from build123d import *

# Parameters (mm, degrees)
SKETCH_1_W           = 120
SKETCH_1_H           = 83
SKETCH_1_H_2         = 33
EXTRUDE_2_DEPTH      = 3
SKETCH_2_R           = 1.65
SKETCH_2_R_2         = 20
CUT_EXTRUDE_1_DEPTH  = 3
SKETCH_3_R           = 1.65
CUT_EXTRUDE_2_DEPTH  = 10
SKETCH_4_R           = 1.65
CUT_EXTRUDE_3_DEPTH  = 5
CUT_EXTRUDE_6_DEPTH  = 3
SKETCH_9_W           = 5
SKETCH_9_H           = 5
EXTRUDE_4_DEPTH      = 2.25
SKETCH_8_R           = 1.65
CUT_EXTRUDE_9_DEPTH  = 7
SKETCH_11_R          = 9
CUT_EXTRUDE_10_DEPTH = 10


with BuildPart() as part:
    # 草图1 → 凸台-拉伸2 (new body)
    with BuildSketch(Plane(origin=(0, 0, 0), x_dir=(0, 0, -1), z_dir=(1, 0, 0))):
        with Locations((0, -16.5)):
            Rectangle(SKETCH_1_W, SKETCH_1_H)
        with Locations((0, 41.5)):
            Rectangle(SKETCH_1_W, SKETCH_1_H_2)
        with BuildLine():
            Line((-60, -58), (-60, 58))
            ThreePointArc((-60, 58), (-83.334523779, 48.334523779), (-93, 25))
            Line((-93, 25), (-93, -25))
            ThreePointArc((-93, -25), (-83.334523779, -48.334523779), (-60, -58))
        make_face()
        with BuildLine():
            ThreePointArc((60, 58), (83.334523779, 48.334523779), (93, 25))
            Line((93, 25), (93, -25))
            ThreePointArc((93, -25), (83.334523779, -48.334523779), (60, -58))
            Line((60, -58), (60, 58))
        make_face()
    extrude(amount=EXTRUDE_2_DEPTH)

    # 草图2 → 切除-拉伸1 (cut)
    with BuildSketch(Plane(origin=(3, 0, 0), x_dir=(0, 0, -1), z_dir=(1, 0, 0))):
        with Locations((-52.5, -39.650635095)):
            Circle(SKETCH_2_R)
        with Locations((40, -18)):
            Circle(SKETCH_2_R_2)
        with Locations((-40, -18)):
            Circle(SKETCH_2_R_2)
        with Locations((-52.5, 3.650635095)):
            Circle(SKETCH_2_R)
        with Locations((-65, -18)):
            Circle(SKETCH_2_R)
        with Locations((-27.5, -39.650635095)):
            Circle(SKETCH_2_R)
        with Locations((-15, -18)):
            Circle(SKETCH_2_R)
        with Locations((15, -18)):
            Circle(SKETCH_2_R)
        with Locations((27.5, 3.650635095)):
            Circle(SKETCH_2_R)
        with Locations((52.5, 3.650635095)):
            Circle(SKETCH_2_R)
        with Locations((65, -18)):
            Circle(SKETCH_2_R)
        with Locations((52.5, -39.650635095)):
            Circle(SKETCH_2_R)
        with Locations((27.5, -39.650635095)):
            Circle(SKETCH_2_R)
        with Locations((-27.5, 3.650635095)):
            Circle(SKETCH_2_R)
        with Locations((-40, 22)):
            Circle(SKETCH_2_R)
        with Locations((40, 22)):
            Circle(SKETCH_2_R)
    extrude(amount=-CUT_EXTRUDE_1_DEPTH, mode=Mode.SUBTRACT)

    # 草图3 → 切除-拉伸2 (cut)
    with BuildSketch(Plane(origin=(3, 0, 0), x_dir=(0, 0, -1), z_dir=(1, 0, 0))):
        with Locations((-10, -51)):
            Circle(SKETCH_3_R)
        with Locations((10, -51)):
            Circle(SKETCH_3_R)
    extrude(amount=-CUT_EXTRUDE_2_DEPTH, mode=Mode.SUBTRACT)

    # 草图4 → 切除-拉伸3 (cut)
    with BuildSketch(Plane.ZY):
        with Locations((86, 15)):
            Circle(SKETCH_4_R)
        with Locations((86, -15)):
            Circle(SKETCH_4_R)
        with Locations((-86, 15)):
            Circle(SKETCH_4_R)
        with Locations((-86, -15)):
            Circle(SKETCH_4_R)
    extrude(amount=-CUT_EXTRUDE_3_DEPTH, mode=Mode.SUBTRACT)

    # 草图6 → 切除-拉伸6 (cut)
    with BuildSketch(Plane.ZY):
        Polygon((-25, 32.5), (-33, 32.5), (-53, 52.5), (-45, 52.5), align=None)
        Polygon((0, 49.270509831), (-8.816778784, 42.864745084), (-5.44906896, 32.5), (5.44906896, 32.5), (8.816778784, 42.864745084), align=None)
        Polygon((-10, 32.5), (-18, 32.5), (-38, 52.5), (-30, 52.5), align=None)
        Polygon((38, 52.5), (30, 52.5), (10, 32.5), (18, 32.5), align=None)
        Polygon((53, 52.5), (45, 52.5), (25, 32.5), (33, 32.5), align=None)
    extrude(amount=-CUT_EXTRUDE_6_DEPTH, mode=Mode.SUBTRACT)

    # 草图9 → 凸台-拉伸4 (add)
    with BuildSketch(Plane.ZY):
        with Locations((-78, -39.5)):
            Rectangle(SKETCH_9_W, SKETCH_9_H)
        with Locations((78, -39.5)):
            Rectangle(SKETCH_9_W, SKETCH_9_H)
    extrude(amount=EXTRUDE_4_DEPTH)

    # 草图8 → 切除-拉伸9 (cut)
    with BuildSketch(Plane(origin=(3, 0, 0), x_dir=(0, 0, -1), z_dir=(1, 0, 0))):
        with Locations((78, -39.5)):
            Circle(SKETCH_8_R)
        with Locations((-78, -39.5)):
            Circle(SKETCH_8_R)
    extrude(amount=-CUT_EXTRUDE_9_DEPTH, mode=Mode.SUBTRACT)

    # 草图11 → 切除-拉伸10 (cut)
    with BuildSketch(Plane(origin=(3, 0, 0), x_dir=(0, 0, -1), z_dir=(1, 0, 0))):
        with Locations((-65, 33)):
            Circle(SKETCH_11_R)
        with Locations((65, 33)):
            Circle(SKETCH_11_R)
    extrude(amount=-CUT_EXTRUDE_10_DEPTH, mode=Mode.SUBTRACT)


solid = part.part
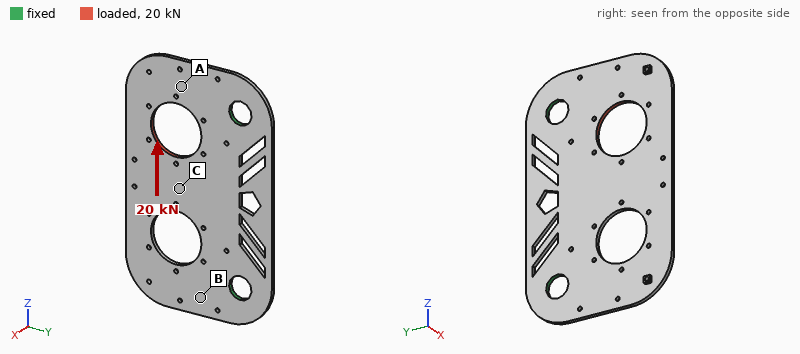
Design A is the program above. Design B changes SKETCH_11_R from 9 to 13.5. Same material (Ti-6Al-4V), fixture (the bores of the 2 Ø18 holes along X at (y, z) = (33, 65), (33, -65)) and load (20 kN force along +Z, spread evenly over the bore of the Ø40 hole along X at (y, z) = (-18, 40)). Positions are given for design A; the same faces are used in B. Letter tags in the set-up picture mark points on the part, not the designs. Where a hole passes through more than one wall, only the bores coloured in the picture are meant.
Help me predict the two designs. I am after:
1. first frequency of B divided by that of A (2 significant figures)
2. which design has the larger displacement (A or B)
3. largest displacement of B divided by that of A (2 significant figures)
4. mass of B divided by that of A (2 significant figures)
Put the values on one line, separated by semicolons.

1.1; A; 0.88; 0.96
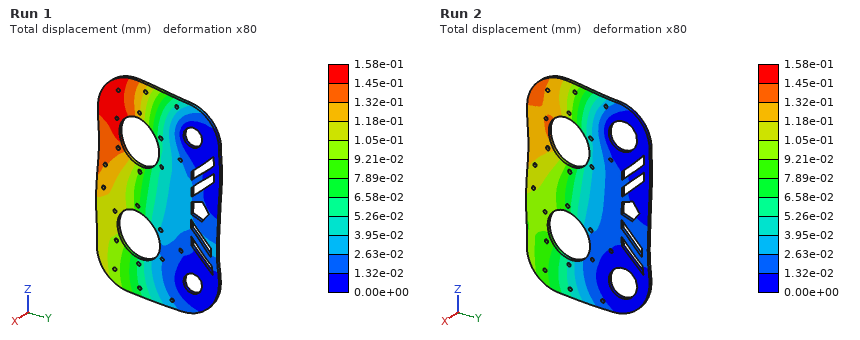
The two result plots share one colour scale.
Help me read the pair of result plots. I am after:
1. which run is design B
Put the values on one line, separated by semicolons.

Run 2
